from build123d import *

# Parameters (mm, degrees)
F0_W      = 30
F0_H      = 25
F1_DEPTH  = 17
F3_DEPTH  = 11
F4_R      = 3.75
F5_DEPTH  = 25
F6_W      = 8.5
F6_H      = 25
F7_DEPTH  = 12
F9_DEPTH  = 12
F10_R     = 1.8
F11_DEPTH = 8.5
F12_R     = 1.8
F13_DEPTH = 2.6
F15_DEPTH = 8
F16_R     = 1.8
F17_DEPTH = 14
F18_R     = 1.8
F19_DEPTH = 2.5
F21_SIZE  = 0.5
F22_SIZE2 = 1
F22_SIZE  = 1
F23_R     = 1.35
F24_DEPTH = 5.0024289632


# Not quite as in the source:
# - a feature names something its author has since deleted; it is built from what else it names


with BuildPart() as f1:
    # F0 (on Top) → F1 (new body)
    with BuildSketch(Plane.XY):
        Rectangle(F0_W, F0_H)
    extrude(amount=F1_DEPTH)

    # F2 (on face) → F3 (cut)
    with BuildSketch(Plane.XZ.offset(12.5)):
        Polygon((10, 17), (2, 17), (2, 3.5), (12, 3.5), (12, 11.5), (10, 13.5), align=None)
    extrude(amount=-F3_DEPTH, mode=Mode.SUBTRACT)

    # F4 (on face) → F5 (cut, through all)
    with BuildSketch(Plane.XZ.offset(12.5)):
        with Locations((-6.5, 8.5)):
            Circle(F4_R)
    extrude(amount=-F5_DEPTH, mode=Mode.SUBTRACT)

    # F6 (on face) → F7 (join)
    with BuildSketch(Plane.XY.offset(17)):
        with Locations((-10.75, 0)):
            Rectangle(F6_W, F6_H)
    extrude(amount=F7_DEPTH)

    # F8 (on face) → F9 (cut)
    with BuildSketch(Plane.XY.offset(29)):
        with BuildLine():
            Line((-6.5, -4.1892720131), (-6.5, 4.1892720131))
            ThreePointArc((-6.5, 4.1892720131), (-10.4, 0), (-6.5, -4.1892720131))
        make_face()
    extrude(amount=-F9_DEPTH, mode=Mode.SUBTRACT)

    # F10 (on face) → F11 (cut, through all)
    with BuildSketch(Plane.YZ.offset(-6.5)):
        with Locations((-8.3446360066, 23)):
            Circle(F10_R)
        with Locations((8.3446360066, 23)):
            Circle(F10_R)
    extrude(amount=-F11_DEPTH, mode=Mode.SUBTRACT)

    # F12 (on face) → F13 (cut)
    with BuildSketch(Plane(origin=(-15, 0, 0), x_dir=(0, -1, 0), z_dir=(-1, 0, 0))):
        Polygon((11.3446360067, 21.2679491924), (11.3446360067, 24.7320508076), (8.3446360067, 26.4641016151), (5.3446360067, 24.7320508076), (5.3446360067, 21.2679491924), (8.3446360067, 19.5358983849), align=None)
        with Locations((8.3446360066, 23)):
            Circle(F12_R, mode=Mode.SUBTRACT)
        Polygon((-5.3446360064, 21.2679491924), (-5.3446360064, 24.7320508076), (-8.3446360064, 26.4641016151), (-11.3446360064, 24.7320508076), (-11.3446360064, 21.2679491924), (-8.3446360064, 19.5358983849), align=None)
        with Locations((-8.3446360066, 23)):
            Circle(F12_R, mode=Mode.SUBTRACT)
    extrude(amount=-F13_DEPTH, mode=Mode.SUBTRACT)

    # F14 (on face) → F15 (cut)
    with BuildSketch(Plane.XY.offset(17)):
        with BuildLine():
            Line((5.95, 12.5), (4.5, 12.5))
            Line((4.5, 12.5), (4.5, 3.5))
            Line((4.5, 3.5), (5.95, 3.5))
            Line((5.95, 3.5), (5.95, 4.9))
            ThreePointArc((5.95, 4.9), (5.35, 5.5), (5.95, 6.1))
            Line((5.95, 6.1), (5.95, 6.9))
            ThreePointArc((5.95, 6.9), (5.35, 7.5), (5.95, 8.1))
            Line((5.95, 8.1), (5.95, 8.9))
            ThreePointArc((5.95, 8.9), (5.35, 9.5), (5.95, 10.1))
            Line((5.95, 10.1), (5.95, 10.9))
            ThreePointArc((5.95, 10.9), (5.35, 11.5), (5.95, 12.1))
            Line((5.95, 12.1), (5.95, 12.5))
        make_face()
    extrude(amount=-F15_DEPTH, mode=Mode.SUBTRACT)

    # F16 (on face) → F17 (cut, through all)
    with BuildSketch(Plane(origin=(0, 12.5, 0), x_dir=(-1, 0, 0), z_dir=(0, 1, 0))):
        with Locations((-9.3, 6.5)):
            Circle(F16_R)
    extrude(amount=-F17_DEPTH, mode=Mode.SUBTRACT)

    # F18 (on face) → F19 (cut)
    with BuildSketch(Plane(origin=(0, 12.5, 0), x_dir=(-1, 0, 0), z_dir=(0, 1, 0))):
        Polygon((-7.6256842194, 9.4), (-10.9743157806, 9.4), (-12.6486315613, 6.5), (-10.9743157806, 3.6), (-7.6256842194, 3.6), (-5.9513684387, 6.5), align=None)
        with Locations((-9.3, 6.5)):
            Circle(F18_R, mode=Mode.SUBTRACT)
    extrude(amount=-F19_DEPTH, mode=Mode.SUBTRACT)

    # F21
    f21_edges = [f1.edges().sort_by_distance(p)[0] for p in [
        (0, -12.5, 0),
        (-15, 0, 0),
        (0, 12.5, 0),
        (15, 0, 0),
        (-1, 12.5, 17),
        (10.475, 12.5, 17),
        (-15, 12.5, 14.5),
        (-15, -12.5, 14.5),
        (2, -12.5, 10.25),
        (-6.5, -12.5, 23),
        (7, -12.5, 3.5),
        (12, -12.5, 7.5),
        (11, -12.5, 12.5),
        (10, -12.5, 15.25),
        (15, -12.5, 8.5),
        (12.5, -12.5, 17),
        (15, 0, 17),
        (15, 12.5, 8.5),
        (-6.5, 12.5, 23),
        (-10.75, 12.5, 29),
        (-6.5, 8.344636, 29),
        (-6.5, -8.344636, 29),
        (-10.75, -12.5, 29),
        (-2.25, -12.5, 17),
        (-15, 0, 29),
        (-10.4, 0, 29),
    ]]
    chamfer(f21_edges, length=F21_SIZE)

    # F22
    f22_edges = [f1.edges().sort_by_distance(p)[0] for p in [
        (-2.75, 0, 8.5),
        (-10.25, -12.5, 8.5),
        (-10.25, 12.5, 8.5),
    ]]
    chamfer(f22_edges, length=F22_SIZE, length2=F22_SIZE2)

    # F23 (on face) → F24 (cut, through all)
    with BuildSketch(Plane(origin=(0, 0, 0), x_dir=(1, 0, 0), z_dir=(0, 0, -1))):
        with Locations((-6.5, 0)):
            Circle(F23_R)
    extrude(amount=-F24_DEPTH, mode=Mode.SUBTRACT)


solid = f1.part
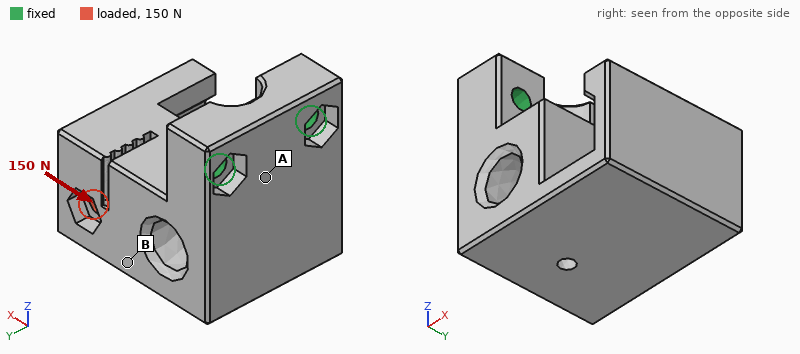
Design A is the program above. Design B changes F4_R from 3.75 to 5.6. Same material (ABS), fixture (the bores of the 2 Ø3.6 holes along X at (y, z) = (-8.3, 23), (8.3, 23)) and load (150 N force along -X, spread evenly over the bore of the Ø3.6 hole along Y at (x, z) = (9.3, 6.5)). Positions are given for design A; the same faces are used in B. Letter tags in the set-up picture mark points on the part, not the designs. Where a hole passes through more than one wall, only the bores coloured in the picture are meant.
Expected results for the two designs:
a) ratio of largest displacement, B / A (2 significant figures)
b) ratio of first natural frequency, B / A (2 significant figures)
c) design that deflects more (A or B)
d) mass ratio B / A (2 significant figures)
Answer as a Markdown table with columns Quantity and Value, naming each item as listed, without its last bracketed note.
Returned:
| Quantity | Value |
|---|---|
| ratio of largest displacement, B / A | 1.3 |
| ratio of first natural frequency, B / A | 0.90 |
| design that deflects more | B |
| mass ratio B / A | 0.89 |
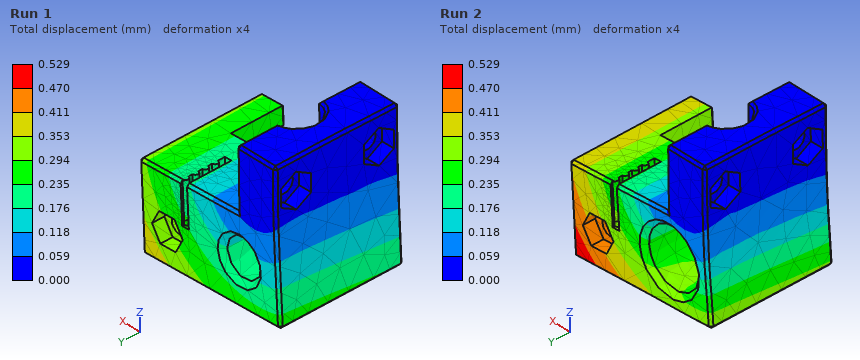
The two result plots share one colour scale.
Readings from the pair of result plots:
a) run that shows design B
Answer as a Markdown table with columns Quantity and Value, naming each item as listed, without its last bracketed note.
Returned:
| Quantity | Value |
|---|---|
| run that shows design B | Run 2 |
